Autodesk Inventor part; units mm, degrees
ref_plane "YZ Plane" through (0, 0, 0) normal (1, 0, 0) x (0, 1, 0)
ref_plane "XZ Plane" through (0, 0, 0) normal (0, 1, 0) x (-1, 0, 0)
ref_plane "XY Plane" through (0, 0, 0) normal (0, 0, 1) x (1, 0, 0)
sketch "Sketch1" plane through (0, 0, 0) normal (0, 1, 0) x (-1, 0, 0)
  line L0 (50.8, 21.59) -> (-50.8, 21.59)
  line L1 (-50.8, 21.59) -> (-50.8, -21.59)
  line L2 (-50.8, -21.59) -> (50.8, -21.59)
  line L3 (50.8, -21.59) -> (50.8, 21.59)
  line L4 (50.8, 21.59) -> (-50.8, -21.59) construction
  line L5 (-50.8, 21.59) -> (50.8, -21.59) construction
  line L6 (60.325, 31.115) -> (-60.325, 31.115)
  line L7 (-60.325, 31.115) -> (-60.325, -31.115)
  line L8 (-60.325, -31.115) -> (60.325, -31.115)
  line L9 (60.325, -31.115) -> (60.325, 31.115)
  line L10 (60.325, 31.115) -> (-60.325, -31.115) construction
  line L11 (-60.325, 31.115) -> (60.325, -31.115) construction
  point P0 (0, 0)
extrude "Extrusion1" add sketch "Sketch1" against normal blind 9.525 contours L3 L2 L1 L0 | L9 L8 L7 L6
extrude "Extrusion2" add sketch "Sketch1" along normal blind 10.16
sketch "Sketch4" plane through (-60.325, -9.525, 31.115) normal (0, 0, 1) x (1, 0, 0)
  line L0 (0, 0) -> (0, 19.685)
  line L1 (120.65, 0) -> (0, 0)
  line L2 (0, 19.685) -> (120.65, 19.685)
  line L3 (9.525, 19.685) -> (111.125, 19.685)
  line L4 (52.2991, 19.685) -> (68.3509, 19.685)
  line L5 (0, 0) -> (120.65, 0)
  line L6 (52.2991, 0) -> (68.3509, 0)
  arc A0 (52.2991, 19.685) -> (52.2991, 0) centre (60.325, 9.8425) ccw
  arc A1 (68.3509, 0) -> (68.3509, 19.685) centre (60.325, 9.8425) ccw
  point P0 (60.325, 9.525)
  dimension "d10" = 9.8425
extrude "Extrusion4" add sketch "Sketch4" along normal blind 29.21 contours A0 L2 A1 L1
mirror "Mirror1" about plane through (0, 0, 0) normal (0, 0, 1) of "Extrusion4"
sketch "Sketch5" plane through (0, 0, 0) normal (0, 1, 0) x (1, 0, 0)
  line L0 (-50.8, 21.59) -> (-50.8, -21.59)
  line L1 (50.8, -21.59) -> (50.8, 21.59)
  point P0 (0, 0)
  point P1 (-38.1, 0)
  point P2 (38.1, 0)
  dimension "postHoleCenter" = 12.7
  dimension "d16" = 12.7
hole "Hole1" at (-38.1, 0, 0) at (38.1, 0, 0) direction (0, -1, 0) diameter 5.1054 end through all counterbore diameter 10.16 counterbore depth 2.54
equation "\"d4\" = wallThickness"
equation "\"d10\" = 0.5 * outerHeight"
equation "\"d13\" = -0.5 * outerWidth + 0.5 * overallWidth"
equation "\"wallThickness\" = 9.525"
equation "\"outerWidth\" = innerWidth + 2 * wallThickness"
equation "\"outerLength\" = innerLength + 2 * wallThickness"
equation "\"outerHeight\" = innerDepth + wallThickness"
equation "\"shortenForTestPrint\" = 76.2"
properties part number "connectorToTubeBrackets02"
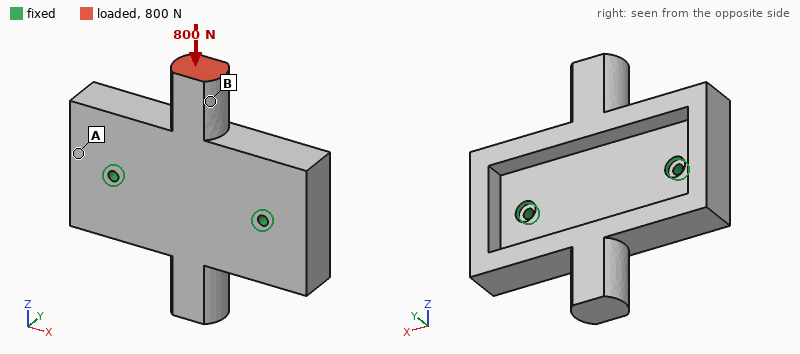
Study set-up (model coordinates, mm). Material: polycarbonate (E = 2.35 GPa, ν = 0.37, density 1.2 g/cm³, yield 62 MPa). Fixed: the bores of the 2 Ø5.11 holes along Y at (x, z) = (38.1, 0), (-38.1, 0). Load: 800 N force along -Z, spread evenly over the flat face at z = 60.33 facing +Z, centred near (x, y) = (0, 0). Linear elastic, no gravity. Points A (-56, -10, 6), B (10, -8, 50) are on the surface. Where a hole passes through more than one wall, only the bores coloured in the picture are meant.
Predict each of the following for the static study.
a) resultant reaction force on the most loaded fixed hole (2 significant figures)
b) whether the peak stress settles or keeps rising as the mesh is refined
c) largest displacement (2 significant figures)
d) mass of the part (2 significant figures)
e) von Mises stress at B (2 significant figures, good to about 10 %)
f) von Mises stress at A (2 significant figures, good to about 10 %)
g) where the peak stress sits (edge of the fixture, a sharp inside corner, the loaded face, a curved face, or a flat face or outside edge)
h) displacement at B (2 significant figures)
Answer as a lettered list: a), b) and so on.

a) 410 N
b) keeps rising
c) 0.65 mm
d) 150 g
e) 1.8 MPa
f) 0.96 MPa
g) edge of the fixture
h) 0.48 mm
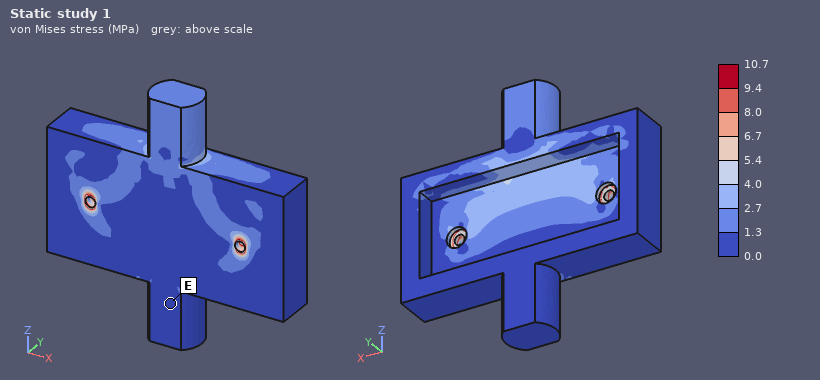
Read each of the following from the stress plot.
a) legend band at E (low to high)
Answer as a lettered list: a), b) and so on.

a) 0.0 to 1.3 MPa
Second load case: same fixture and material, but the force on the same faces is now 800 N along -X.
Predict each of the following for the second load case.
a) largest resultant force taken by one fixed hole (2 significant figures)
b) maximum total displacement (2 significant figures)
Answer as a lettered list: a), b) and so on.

a) 750 N
b) 0.53 mm
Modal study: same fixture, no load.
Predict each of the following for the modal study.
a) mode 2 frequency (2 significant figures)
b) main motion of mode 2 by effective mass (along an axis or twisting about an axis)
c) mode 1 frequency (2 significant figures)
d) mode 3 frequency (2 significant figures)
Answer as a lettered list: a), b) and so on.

a) 780 Hz
b) along Y
c) 400 Hz
d) 1200 Hz
